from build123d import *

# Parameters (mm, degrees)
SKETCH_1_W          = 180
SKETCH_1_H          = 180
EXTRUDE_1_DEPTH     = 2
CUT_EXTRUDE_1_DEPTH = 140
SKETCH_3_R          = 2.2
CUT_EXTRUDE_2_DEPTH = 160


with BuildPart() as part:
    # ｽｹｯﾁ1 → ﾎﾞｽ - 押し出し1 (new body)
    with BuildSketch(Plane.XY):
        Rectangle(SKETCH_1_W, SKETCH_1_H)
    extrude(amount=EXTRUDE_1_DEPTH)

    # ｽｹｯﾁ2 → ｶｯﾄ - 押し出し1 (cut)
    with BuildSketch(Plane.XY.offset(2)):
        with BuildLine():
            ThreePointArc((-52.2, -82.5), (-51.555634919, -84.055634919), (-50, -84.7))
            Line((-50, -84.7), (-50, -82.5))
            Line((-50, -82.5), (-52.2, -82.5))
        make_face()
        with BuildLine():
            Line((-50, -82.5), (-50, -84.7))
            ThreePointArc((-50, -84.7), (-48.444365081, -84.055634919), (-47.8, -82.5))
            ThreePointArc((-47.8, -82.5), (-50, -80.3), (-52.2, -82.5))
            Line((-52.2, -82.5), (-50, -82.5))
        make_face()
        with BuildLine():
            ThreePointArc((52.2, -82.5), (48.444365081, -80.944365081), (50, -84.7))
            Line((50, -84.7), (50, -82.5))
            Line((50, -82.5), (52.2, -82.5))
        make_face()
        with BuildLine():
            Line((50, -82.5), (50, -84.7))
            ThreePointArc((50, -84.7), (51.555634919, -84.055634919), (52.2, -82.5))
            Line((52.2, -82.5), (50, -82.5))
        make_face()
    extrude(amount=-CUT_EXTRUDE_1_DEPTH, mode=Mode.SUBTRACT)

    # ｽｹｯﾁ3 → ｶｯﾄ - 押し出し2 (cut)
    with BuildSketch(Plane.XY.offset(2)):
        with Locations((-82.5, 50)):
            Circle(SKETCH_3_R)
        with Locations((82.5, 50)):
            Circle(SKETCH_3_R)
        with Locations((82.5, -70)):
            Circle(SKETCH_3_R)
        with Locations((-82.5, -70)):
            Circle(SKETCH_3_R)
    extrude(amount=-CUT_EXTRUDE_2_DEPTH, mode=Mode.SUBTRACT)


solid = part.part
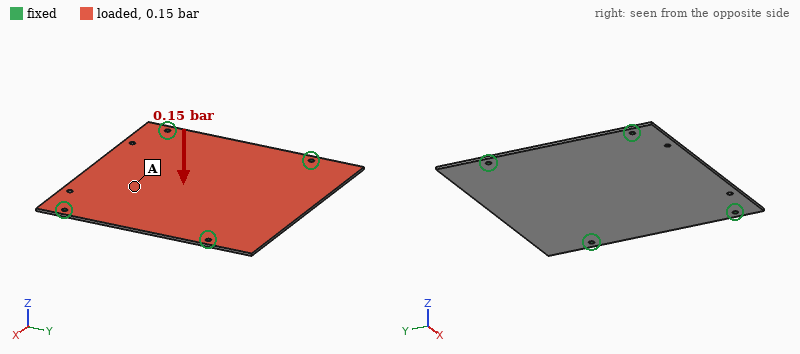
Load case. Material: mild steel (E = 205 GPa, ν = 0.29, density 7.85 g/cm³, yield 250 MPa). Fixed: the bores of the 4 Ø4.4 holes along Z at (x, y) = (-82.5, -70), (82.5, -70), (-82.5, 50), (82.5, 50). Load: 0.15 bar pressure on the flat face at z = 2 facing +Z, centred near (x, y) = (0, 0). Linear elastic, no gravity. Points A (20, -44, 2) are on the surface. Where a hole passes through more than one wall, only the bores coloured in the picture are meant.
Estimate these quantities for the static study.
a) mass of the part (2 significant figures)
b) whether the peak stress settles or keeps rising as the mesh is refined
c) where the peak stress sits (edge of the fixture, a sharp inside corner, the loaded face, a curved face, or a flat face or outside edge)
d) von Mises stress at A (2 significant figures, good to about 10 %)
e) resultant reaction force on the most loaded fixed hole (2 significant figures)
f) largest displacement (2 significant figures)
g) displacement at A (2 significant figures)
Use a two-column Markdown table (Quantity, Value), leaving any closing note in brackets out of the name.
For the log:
| Quantity | Value |
|---|---|
| mass of the part | 510 g |
| whether the peak stress settles or keeps rising as the mesh is refined | keeps rising |
| where the peak stress sits | edge of the fixture |
| von Mises stress at A | 25 MPa |
| resultant reaction force on the most loaded fixed hole | 140 N |
| largest displacement | 0.37 mm |
| displacement at A | 0.31 mm |
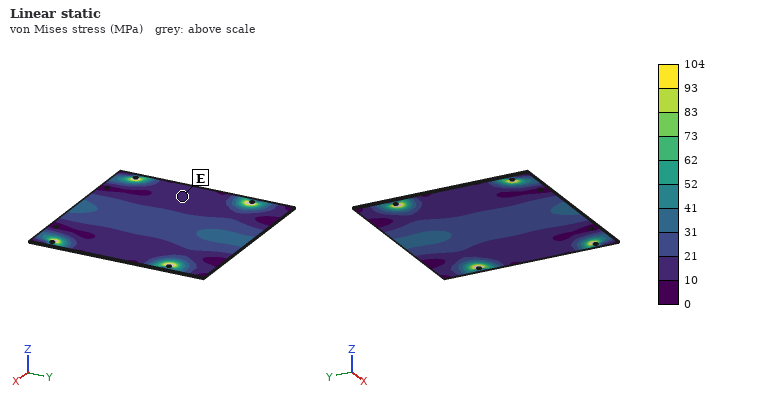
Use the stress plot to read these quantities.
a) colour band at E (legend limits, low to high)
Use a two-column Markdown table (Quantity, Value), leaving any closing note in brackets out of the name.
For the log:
| Quantity | Value |
|---|---|
| colour band at E | 10 to 21 MPa |
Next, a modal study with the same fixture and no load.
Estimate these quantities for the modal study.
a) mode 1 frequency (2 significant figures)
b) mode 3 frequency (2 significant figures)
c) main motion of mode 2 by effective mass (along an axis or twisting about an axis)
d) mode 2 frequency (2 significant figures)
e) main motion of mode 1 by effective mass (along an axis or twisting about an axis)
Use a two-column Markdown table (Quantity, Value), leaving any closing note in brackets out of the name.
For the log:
| Quantity | Value |
|---|---|
| mode 1 frequency | 300 Hz |
| mode 3 frequency | 540 Hz |
| main motion of mode 2 by effective mass | twisting about X |
| mode 2 frequency | 380 Hz |
| main motion of mode 1 by effective mass | along Z |
